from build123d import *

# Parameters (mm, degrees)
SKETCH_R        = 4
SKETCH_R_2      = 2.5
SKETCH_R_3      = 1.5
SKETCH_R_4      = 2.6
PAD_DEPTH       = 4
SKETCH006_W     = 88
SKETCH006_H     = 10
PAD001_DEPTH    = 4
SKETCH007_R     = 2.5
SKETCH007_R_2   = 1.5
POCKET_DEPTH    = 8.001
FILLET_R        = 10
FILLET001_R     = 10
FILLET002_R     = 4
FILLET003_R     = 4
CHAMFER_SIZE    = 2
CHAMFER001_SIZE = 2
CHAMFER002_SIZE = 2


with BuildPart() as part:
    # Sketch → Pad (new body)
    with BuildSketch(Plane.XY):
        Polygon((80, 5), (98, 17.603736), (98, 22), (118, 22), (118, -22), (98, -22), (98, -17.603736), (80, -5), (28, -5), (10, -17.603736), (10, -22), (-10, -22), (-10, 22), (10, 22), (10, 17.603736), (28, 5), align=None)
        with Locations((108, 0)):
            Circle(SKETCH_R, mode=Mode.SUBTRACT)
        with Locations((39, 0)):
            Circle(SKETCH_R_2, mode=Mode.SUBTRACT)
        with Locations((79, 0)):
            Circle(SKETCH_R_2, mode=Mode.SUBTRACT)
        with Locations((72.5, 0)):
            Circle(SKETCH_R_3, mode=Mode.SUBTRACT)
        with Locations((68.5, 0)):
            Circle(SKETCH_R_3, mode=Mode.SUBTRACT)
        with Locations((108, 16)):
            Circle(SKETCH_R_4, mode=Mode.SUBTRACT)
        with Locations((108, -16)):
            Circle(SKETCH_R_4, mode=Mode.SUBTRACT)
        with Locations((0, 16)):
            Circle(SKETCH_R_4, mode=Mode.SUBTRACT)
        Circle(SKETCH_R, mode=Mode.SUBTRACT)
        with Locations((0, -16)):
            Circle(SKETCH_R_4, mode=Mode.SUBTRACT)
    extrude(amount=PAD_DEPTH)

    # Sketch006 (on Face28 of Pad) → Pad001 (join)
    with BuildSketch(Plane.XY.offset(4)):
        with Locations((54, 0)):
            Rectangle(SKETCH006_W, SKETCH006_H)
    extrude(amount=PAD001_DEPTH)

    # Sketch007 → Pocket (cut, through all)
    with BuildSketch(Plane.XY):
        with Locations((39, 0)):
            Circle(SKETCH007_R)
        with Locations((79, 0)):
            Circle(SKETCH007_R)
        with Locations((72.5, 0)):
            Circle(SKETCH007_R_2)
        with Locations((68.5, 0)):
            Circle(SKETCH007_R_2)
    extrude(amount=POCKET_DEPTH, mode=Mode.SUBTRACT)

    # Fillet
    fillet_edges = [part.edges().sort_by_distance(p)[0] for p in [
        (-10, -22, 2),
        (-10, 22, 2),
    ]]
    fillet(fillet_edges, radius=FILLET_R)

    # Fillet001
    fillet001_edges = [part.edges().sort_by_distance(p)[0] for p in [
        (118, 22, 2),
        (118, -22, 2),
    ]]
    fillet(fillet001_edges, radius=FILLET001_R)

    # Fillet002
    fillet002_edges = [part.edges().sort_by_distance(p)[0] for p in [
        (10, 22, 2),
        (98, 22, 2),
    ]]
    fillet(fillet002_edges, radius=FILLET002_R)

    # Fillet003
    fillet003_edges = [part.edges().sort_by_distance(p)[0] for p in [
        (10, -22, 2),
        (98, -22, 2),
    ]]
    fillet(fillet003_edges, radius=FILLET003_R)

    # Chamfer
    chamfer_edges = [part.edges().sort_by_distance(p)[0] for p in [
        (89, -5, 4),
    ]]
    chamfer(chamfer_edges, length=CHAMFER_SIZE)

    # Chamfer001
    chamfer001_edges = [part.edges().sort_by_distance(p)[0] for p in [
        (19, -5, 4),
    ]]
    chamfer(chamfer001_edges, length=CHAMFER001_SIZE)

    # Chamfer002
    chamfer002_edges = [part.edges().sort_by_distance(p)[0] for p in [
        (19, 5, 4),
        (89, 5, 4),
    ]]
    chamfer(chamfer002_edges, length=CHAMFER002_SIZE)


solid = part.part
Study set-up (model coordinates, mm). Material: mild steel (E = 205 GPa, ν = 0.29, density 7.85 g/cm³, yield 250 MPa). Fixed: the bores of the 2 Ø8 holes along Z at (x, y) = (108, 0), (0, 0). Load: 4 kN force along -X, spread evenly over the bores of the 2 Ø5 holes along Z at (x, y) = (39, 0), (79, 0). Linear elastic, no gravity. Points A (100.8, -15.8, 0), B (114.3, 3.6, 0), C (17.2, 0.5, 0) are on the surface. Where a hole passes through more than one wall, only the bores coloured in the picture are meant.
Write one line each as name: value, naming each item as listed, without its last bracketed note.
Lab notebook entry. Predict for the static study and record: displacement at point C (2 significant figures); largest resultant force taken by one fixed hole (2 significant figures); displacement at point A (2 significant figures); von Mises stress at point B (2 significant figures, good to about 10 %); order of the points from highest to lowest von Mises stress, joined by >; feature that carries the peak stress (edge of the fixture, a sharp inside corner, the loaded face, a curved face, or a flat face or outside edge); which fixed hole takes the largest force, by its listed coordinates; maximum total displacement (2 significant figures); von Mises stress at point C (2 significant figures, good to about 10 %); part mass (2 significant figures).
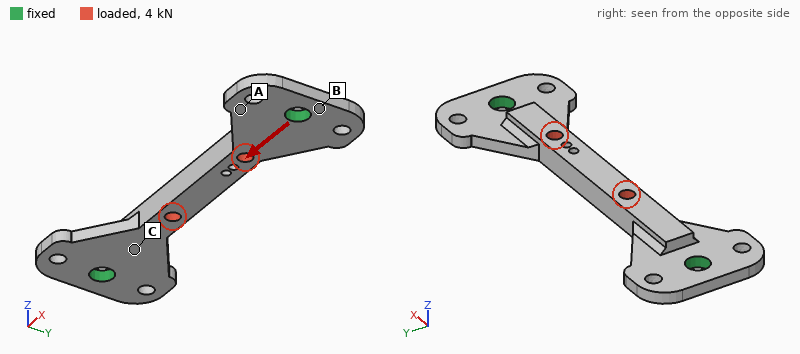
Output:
displacement at point C: 2.2 µm
largest resultant force taken by one fixed hole: 2.2 kN
displacement at point A: 1.3 µm
von Mises stress at point B: 8.8 MPa
order of the points from highest to lowest von Mises stress, joined by >: C > B > A
feature that carries the peak stress: the loaded face
which fixed hole takes the largest force, by its listed coordinates: (108, 0)
maximum total displacement: 7.5 µm
von Mises stress at point C: 25 MPa
part mass: 110 g
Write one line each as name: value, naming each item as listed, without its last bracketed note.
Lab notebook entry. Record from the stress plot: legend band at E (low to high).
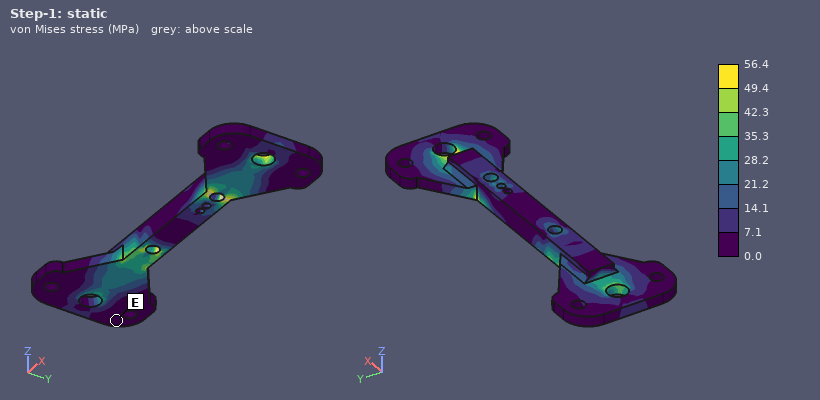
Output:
legend band at E: 0.0 to 7.1 MPa
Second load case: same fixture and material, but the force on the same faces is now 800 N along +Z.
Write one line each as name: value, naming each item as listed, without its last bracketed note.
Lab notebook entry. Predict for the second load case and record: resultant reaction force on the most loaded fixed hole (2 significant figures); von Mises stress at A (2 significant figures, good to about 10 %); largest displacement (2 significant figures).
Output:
resultant reaction force on the most loaded fixed hole: 960 N
von Mises stress at A: 24 MPa
largest displacement: 55 µm
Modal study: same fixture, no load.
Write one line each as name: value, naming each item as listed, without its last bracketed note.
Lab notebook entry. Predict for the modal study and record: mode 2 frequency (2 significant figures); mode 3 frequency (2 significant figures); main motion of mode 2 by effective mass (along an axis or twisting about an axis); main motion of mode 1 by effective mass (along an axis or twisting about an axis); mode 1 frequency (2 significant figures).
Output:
mode 2 frequency: 6100 Hz
mode 3 frequency: 7700 Hz
main motion of mode 2 by effective mass: along Y
main motion of mode 1 by effective mass: along Z
mode 1 frequency: 3100 Hz
